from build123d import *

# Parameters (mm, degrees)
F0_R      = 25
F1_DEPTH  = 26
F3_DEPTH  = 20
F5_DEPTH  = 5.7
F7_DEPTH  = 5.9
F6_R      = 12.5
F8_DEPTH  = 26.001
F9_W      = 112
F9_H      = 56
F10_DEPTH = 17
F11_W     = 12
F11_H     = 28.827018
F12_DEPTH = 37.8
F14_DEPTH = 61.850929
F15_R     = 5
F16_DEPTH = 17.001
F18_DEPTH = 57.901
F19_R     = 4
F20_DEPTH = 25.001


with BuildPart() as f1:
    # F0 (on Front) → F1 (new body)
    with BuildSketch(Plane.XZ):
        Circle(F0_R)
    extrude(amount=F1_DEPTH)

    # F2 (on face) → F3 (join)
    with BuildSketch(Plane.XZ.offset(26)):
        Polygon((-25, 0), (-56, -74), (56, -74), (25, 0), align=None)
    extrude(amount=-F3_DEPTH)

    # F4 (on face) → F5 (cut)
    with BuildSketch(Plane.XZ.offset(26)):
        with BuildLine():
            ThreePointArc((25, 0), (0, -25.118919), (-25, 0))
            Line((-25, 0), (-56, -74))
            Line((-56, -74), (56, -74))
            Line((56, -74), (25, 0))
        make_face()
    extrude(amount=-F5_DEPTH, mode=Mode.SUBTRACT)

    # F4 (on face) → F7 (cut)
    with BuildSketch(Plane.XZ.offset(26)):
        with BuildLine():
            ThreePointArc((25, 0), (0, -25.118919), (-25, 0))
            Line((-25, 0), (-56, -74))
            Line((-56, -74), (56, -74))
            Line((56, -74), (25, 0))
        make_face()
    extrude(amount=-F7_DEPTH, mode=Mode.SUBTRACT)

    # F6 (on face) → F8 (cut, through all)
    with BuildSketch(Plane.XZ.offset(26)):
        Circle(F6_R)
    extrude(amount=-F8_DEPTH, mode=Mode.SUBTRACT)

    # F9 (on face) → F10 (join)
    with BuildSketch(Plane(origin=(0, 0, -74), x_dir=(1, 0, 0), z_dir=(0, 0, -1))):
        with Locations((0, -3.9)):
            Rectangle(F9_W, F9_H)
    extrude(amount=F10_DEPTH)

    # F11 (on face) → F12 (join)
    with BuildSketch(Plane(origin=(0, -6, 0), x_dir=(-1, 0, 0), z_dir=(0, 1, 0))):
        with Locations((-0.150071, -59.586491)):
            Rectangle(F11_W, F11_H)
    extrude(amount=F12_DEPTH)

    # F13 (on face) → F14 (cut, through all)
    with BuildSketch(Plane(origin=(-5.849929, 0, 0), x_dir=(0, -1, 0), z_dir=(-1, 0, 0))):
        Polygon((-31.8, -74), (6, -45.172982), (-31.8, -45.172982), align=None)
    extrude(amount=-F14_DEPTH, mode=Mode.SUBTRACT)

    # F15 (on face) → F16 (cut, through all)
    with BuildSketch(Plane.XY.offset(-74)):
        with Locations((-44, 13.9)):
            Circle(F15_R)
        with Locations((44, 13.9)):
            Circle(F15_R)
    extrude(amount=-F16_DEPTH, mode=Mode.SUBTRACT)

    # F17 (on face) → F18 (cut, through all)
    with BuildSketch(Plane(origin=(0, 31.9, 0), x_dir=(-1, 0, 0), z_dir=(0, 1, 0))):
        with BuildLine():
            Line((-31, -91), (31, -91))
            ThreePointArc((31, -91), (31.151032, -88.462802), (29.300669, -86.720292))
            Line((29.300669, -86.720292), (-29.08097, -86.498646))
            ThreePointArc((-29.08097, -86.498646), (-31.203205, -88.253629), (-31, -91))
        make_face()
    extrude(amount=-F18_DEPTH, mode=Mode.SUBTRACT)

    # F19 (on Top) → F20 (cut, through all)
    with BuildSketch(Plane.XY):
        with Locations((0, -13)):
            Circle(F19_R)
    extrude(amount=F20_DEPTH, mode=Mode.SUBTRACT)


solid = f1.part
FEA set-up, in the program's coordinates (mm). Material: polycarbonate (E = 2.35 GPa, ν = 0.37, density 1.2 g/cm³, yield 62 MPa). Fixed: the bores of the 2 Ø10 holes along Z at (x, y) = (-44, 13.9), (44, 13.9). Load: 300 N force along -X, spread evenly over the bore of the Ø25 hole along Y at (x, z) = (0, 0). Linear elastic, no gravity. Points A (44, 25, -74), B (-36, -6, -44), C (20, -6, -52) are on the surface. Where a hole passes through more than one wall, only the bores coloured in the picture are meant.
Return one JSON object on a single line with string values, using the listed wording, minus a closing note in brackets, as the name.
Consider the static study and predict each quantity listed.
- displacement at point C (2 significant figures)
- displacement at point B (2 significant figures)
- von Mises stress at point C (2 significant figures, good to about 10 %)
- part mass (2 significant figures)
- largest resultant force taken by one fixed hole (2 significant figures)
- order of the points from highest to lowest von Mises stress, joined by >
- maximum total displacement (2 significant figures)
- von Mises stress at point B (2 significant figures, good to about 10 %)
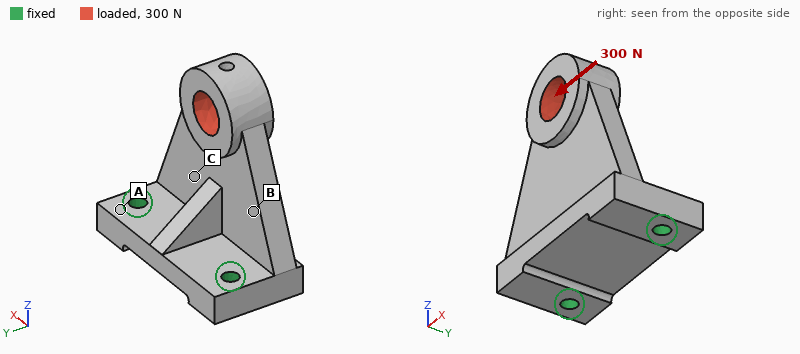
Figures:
{"displacement at point C": "0.050 mm", "displacement at point B": "0.073 mm", "von Mises stress at point C": "0.74 MPa", "part mass": "240 g", "largest resultant force taken by one fixed hole": "330 N", "order of the points from highest to lowest von Mises stress, joined by >": "B > C > A", "maximum total displacement": "0.18 mm", "von Mises stress at point B": "1.1 MPa"}
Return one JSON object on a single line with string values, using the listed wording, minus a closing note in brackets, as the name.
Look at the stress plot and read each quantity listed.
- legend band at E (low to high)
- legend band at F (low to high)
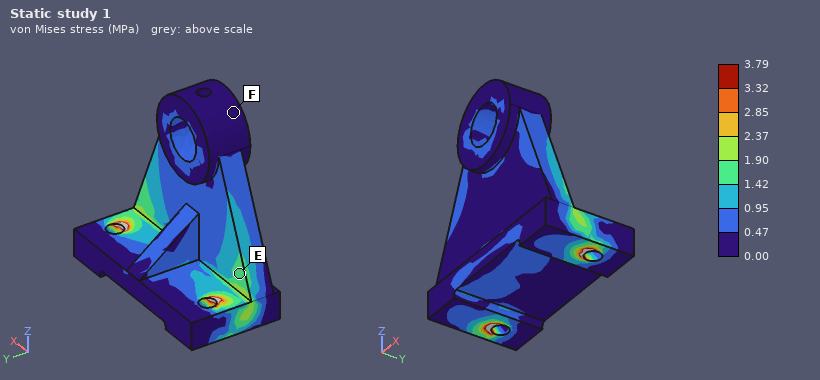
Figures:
{"legend band at E": "1.42 to 1.90 MPa", "legend band at F": "0.00 to 0.47 MPa"}
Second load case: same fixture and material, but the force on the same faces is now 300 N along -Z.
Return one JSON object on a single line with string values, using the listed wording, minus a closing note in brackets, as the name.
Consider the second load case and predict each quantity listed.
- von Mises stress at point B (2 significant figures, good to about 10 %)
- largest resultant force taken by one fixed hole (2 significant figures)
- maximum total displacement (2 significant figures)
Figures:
{"von Mises stress at point B": "0.38 MPa", "largest resultant force taken by one fixed hole": "150 N", "maximum total displacement": "0.17 mm"}
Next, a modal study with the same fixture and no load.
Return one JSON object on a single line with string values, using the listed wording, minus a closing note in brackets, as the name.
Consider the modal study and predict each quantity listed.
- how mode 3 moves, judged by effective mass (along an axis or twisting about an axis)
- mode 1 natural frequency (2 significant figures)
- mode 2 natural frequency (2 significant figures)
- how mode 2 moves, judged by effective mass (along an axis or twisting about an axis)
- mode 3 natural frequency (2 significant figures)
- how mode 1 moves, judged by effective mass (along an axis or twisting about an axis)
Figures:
{"how mode 3 moves, judged by effective mass": "along Z", "mode 1 natural frequency": "320 Hz", "mode 2 natural frequency": "880 Hz", "how mode 2 moves, judged by effective mass": "along X", "mode 3 natural frequency": "1100 Hz", "how mode 1 moves, judged by effective mass": "along Y"}
